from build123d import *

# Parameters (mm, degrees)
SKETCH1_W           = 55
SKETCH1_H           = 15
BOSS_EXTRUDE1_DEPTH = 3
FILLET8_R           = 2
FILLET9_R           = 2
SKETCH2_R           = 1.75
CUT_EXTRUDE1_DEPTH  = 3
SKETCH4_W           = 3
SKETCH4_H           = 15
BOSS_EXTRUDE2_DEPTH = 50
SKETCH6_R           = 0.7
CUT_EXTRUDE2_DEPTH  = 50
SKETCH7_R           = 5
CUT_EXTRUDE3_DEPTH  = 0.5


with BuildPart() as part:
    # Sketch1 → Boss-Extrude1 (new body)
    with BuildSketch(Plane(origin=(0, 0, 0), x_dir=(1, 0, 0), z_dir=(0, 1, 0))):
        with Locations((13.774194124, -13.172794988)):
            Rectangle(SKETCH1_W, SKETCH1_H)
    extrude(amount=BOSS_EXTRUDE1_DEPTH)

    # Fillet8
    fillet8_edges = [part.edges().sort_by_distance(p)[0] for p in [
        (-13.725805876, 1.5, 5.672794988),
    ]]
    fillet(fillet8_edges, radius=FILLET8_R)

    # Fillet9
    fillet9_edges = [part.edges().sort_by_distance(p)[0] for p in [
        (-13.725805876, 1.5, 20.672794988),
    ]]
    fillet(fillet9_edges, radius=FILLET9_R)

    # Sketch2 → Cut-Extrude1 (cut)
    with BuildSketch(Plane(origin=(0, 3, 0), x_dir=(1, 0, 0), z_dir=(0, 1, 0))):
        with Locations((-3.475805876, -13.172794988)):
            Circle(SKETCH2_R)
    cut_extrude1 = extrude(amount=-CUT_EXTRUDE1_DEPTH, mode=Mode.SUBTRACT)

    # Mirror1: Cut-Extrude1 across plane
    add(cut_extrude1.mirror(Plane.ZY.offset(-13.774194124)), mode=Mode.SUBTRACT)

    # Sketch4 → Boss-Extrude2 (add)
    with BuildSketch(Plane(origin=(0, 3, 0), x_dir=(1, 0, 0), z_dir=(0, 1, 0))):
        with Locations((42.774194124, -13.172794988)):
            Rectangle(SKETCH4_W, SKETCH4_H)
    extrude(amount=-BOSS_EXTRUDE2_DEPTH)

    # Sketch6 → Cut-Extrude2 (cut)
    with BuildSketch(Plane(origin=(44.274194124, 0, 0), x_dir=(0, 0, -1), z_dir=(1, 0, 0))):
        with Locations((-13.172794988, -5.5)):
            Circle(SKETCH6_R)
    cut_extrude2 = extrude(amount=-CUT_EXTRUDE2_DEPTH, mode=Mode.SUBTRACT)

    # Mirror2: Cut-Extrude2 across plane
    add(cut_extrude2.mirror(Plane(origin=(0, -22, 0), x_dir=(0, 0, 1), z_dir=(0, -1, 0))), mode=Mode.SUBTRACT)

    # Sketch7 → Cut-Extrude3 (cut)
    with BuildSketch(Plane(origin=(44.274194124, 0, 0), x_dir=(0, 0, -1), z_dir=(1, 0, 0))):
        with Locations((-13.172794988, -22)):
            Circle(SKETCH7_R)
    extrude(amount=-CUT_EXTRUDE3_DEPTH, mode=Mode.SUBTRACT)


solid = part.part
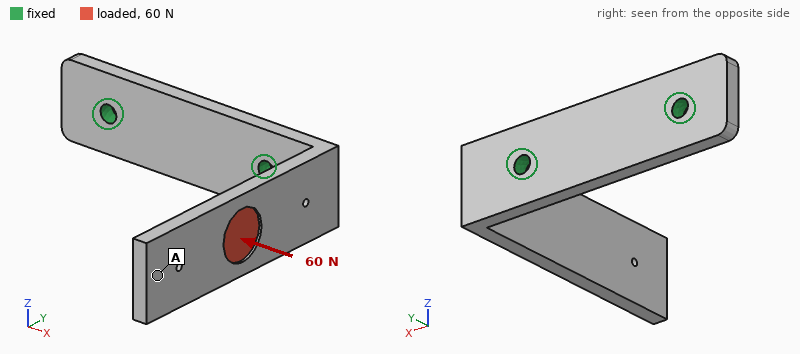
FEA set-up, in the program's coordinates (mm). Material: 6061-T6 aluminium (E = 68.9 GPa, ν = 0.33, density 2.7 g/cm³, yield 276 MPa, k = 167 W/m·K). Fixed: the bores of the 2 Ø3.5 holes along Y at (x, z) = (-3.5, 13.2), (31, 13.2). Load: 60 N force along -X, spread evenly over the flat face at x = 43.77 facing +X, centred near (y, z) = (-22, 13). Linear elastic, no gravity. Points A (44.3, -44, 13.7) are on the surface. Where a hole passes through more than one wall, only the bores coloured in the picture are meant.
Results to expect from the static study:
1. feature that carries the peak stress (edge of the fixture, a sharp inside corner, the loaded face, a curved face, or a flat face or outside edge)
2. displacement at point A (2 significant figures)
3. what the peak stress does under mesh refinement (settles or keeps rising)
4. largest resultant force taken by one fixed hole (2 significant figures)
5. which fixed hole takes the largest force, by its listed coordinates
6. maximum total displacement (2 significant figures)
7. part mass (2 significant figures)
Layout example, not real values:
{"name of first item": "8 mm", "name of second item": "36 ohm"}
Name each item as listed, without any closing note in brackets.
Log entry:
{"feature that carries the peak stress": "edge of the fixture", "displacement at point A": "0.55 mm", "what the peak stress does under mesh refinement": "keeps rising", "largest resultant force taken by one fixed hole": "56 N", "which fixed hole takes the largest force, by its listed coordinates": "(31, 13.2)", "maximum total displacement": "0.59 mm", "part mass": "12 g"}
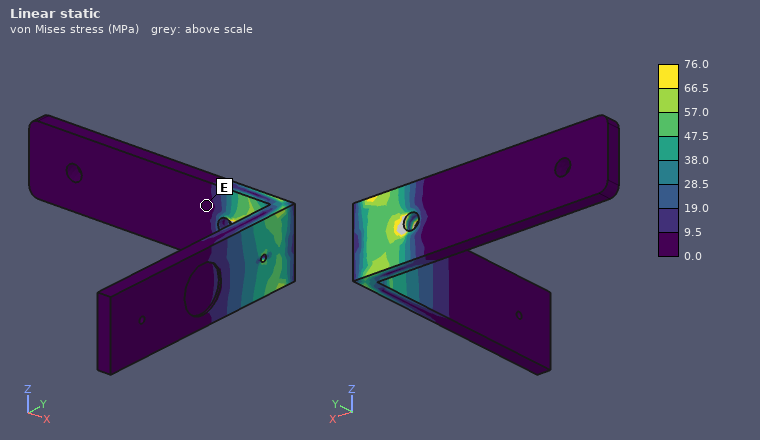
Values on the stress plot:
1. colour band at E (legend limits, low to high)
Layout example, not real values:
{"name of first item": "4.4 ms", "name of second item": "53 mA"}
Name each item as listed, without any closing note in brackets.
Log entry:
{"colour band at E": "0.0 to 9.5 MPa"}
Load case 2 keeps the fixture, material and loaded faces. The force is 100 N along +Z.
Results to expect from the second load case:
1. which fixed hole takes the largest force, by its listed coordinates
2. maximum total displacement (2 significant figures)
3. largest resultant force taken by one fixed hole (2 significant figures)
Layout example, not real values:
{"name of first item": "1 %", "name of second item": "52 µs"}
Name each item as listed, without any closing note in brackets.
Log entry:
{"which fixed hole takes the largest force, by its listed coordinates": "(31, 13.2)", "maximum total displacement": "0.34 mm", "largest resultant force taken by one fixed hole": "120 N"}
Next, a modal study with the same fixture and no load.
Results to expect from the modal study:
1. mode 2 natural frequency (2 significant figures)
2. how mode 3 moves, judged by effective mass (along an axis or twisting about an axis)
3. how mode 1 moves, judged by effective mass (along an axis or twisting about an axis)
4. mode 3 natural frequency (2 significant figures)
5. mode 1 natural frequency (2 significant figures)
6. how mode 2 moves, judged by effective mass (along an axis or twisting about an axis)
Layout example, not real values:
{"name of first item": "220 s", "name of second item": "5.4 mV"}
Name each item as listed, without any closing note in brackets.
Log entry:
{"mode 2 natural frequency": "1300 Hz", "how mode 3 moves, judged by effective mass": "along Y", "how mode 1 moves, judged by effective mass": "along X", "mode 3 natural frequency": "4300 Hz", "mode 1 natural frequency": "770 Hz", "how mode 2 moves, judged by effective mass": "along Z"}
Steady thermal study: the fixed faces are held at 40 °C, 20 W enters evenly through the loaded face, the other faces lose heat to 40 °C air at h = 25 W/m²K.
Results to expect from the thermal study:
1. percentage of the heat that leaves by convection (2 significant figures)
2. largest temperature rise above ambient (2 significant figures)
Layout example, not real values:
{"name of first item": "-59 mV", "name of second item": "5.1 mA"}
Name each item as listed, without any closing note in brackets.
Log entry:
{"percentage of the heat that leaves by convection": "15 %", "largest temperature rise above ambient": "83 K"}
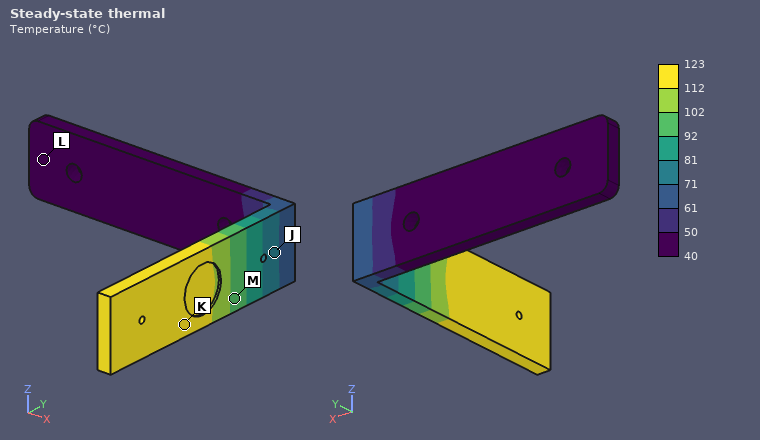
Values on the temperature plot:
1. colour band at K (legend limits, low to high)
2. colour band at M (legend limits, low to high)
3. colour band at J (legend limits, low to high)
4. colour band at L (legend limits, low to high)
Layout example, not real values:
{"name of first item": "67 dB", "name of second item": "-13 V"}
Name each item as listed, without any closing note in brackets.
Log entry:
{"colour band at K": "112 to 123 °C", "colour band at M": "92 to 102 °C", "colour band at J": "71 to 81 °C", "colour band at L": "40 to 50 °C"}
